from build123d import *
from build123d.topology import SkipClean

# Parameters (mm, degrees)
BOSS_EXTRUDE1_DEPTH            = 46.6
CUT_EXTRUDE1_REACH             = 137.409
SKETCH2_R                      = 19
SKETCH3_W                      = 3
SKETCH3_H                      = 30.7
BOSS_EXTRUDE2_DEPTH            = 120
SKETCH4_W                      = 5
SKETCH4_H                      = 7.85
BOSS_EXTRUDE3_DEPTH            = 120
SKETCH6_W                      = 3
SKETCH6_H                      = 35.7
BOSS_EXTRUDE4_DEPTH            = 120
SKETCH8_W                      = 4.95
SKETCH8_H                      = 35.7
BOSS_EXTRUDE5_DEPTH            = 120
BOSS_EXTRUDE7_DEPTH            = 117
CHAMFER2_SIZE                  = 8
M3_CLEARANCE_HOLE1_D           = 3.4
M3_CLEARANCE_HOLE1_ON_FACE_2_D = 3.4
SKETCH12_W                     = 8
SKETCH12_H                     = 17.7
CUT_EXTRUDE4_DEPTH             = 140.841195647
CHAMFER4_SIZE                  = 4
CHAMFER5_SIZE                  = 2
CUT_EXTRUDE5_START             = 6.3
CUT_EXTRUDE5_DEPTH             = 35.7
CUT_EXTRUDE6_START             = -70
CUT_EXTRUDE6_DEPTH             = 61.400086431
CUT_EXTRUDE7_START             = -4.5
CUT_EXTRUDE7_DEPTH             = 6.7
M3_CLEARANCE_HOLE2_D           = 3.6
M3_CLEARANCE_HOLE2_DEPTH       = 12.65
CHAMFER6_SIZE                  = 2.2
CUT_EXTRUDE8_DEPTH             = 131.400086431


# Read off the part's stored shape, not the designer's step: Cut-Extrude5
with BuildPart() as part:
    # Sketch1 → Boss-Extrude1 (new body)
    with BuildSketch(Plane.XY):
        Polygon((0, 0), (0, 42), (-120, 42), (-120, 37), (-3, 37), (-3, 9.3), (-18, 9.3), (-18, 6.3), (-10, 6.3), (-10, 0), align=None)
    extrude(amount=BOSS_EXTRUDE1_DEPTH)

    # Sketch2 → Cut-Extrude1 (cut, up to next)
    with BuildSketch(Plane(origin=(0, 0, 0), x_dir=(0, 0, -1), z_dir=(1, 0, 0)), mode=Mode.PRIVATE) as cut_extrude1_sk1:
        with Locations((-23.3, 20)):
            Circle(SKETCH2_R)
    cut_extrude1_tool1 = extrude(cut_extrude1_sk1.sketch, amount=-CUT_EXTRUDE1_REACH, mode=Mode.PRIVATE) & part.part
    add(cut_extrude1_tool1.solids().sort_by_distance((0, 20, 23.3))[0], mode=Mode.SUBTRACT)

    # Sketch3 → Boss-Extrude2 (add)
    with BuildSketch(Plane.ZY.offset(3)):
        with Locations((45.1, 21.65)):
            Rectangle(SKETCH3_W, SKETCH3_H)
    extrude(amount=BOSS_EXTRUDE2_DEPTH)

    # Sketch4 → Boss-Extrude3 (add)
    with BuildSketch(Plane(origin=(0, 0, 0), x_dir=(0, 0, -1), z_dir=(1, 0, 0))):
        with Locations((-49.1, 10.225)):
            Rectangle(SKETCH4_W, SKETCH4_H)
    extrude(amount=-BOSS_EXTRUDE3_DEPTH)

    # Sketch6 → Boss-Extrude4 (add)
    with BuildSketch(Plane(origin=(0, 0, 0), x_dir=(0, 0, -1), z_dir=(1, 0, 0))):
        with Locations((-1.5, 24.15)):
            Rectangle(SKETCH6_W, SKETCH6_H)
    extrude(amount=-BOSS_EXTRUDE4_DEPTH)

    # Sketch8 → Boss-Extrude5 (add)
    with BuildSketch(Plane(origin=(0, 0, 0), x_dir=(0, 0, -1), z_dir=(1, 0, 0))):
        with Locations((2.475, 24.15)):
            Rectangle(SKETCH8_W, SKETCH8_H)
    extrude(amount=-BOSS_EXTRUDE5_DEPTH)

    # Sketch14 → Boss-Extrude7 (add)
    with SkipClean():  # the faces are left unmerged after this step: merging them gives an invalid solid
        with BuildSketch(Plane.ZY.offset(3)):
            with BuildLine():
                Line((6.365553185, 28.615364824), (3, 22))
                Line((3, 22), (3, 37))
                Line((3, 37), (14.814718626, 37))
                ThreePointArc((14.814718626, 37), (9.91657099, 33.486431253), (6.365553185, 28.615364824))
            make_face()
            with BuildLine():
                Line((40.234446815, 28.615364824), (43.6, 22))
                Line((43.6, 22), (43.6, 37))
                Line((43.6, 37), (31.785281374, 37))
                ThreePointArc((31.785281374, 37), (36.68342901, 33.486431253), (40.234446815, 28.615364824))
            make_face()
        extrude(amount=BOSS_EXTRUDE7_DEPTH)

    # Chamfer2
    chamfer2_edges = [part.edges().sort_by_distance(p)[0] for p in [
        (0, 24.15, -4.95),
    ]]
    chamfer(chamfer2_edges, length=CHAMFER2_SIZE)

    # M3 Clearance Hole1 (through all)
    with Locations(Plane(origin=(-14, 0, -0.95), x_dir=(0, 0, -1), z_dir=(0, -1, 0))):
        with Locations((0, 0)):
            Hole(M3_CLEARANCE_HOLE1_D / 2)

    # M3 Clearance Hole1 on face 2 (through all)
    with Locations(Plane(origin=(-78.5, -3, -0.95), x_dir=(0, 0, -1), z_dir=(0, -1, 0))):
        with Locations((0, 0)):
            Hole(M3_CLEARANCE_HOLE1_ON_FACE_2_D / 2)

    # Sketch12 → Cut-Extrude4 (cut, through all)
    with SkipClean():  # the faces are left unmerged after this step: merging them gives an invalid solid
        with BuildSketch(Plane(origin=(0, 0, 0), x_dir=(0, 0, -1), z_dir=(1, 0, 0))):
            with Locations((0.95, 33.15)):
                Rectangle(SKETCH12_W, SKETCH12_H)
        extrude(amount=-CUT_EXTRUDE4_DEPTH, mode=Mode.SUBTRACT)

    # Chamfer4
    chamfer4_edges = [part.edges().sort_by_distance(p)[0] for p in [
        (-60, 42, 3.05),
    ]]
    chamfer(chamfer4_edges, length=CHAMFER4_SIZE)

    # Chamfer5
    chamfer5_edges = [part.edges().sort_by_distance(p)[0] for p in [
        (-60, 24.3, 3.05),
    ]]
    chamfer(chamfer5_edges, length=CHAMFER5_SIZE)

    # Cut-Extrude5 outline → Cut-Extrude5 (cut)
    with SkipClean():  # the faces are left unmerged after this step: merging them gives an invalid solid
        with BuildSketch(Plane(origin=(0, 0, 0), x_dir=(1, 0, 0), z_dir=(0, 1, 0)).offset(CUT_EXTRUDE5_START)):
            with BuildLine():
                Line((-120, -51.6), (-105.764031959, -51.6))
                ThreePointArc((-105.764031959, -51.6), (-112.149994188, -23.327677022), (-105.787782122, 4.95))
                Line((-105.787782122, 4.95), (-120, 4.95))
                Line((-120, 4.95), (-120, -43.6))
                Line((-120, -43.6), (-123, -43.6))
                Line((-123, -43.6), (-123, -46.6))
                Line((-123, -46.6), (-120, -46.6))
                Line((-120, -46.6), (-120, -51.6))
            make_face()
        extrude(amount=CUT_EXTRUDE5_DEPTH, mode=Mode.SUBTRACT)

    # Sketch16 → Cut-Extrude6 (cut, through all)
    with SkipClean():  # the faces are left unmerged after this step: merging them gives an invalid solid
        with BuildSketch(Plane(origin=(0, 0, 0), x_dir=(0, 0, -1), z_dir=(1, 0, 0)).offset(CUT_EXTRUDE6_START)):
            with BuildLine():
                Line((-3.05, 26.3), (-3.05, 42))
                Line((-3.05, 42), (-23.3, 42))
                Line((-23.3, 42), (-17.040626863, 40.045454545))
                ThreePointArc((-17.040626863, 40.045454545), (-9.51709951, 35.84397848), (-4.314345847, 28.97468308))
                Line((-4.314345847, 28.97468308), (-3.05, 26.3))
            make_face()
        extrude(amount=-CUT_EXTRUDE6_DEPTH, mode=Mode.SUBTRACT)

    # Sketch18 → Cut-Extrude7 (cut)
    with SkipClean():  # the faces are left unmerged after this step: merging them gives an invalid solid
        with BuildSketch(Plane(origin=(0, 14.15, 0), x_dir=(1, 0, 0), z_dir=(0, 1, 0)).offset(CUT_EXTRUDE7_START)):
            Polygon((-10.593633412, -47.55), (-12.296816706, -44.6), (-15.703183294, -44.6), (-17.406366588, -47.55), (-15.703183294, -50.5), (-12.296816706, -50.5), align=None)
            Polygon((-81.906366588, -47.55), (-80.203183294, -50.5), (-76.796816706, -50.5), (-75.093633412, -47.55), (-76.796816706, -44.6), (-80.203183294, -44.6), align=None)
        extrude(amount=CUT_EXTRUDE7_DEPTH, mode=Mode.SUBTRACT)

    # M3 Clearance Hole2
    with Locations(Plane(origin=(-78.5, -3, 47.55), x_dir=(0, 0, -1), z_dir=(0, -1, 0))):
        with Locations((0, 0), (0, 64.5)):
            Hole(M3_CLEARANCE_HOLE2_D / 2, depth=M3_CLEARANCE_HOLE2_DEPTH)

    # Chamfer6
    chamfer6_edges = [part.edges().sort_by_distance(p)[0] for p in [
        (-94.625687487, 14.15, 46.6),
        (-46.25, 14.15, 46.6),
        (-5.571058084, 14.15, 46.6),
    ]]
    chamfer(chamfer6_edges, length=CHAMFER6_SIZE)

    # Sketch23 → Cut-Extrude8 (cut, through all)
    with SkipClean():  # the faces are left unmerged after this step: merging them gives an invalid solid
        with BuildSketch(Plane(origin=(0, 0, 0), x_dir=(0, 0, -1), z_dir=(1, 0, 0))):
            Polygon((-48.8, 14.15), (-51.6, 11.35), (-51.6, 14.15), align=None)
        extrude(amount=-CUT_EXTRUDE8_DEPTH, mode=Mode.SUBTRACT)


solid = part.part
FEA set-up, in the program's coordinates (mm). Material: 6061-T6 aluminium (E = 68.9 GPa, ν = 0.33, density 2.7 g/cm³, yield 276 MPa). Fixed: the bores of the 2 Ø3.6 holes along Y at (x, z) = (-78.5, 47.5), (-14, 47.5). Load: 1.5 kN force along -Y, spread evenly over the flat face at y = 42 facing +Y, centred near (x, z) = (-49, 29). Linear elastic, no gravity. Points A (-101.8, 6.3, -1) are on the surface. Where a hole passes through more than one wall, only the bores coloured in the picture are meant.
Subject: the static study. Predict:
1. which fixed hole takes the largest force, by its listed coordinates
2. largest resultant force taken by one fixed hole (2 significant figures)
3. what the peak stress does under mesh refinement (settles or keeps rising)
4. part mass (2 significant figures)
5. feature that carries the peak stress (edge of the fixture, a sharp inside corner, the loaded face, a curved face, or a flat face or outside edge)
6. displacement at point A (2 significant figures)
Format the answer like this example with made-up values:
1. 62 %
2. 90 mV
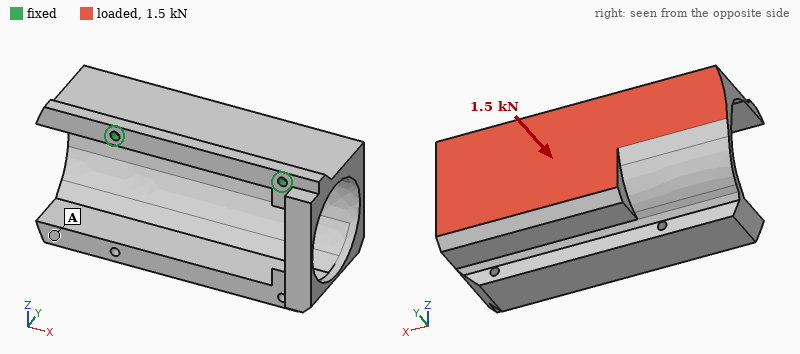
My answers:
1. (-78.5, 47.5)
2. 810 N
3. keeps rising
4. 170 g
5. edge of the fixture
6. 0.79 mm
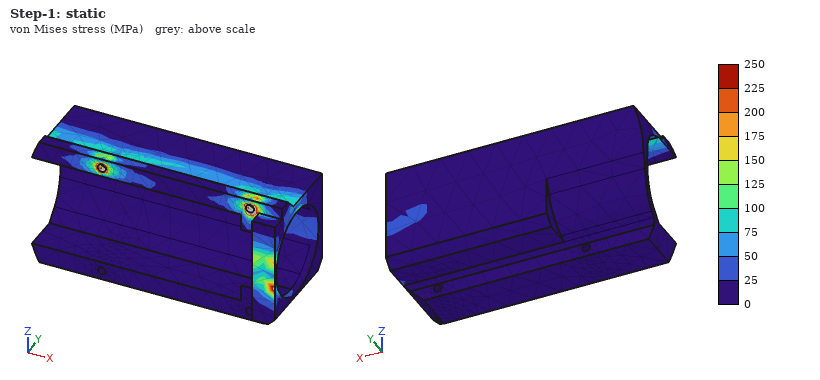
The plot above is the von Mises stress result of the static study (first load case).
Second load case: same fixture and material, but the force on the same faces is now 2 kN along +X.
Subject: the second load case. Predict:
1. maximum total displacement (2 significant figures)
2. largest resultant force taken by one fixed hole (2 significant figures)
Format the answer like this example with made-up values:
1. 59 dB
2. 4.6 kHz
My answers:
1. 0.17 mm
2. 1.6 kN
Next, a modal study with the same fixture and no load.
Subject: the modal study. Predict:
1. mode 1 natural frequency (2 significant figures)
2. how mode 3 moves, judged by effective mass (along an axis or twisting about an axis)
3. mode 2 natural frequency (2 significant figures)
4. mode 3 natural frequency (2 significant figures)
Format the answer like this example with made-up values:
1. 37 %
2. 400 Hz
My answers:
1. 450 Hz
2. along Z
3. 960 Hz
4. 1500 Hz
